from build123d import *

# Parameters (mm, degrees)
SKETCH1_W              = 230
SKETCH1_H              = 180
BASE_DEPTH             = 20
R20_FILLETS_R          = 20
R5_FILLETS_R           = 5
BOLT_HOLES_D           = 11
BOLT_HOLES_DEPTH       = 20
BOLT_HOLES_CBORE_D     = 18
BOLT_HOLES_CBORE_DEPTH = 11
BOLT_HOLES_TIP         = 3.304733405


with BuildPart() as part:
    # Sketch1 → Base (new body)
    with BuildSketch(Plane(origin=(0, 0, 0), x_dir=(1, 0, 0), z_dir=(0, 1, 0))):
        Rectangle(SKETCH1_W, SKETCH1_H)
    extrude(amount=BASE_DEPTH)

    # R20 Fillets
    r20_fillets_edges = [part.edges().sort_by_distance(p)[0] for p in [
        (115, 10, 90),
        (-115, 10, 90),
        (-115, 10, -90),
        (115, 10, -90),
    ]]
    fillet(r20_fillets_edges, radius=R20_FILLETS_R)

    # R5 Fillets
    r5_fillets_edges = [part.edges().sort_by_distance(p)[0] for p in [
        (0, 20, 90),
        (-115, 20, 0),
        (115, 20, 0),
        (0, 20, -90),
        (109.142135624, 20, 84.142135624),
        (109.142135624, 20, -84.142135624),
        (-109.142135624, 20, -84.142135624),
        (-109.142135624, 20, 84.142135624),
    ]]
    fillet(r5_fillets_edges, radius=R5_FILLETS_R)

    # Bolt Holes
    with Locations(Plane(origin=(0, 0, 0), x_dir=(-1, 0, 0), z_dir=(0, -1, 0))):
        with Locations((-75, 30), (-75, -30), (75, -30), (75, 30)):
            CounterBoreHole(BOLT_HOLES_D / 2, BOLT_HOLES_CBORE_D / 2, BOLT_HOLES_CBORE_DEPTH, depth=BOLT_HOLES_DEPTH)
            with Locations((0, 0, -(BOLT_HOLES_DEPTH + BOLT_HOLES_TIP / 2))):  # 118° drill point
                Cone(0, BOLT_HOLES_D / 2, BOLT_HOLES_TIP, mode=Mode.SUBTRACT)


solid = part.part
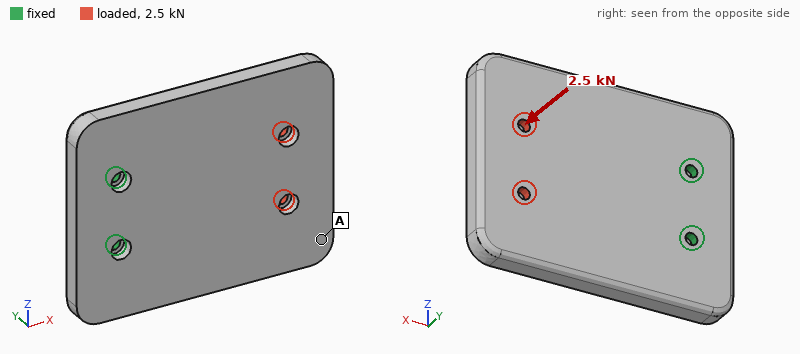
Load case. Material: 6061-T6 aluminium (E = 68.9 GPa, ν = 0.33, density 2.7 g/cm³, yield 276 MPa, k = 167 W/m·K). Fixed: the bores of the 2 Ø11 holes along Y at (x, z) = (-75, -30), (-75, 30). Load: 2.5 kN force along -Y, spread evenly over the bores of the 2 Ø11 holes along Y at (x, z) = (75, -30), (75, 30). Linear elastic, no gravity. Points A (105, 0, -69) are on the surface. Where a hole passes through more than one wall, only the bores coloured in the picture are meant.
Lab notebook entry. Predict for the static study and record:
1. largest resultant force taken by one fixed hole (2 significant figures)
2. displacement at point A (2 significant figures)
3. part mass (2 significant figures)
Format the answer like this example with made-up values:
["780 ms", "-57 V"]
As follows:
["1.6 kN", "0.98 mm", "2.2 kg"]
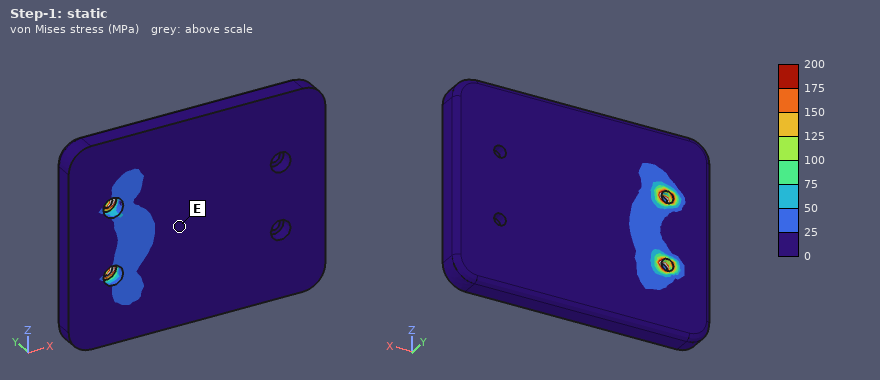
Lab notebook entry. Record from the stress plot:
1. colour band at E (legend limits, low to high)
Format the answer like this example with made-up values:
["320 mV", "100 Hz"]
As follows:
["0 to 25 MPa"]
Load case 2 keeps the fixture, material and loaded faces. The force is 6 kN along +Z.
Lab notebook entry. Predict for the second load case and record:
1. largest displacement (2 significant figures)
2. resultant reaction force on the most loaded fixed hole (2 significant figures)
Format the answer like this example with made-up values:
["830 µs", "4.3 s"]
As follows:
["0.12 mm", "14 kN"]
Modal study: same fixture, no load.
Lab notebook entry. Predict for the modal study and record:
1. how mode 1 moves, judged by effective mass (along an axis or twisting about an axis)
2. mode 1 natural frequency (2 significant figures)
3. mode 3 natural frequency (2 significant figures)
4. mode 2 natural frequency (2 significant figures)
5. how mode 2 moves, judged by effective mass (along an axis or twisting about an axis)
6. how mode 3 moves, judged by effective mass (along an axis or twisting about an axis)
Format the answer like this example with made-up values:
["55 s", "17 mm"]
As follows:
["along Y", "300 Hz", "1300 Hz", "900 Hz", "twisting about X", "along Z"]
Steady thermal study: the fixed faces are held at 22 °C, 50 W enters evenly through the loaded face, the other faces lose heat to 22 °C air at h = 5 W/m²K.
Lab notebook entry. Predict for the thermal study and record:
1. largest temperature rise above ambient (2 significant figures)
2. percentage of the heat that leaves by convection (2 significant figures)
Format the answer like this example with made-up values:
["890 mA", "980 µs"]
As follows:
["18 K", "8.2 %"]
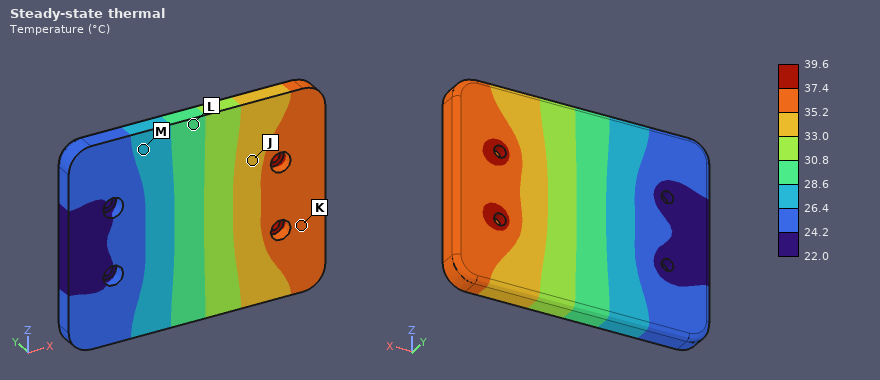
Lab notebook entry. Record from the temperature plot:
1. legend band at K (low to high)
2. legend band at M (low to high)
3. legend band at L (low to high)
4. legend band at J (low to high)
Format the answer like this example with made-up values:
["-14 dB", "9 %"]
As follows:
["35.2 to 37.4 °C", "26.4 to 28.6 °C", "28.6 to 30.8 °C", "33.0 to 35.2 °C"]
